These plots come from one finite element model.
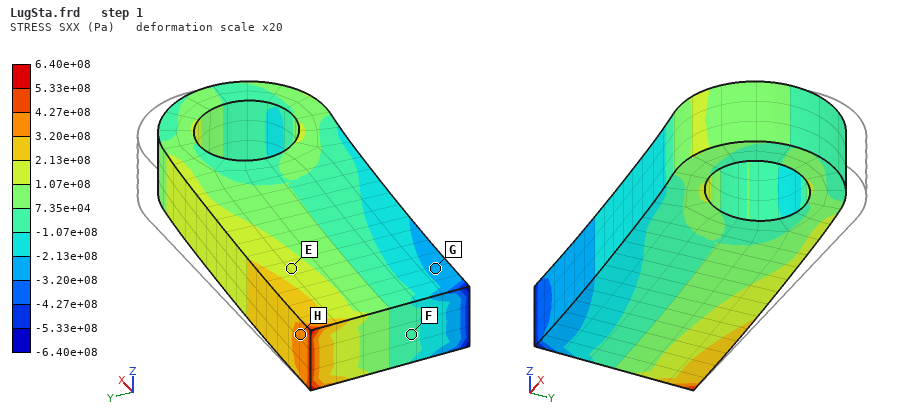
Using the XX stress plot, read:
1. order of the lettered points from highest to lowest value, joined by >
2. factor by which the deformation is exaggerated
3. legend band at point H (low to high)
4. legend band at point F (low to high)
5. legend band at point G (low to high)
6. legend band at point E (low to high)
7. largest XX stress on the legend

H > E > F > G
20
3.20e+08 to 4.27e+08 Pa
-1.07e+08 to 7.35e+04 Pa
-3.20e+08 to -2.13e+08 Pa
1.07e+08 to 2.13e+08 Pa
6.40e+08 Pa
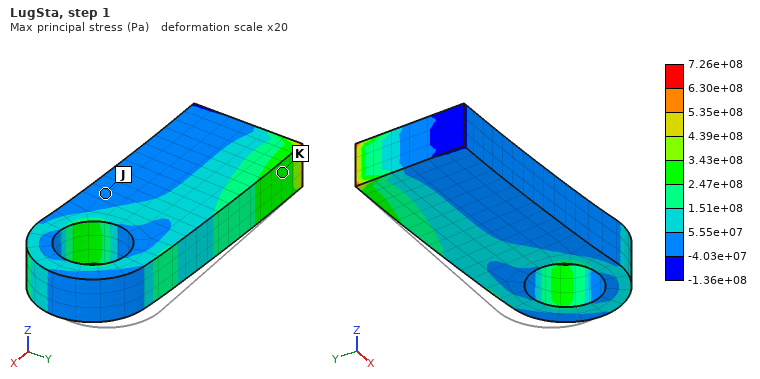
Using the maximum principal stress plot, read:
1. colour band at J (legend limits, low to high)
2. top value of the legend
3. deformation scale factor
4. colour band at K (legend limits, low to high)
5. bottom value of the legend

-4.03e+07 to 5.55e+07 Pa
7.26e+08 Pa
20
2.47e+08 to 3.43e+08 Pa
-1.36e+08 Pa
